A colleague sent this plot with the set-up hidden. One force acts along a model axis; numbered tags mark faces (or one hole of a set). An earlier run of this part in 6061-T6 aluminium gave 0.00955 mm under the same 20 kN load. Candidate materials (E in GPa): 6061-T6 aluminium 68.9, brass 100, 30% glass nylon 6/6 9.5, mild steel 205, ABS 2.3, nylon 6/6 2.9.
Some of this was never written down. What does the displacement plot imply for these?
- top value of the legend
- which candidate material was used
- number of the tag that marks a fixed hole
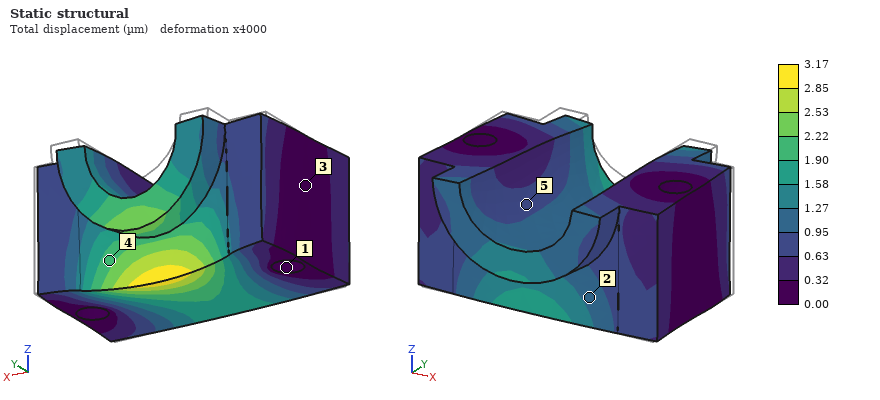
3.17 µm
mild steel
1
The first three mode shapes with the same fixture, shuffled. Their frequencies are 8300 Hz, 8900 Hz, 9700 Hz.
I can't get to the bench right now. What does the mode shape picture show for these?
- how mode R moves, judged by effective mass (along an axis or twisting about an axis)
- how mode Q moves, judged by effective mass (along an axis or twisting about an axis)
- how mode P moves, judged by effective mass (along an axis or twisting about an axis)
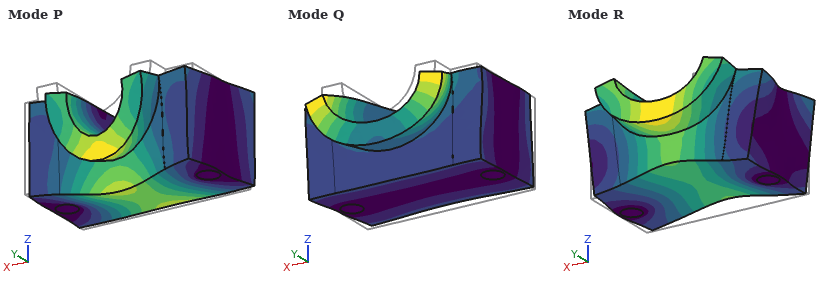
along Z
along Y
along Y
